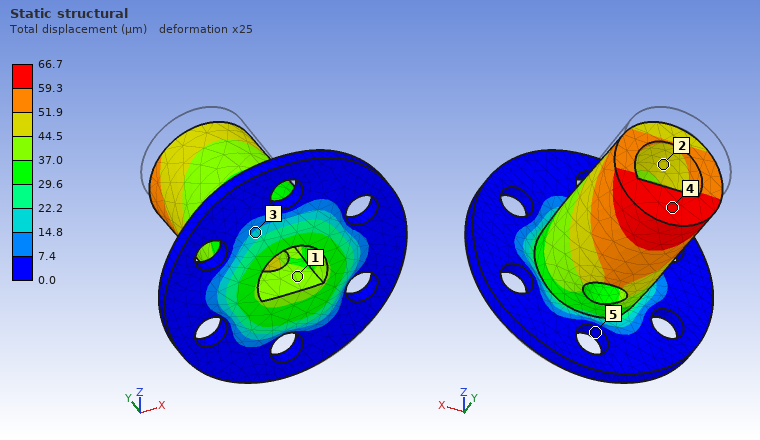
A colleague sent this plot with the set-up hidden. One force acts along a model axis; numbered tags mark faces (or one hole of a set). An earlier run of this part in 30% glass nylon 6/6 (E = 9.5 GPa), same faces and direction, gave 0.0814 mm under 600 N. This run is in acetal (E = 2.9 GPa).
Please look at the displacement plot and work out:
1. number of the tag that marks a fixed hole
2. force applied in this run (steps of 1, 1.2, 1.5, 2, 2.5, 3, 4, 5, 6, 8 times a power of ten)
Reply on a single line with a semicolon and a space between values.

5; 150 N
